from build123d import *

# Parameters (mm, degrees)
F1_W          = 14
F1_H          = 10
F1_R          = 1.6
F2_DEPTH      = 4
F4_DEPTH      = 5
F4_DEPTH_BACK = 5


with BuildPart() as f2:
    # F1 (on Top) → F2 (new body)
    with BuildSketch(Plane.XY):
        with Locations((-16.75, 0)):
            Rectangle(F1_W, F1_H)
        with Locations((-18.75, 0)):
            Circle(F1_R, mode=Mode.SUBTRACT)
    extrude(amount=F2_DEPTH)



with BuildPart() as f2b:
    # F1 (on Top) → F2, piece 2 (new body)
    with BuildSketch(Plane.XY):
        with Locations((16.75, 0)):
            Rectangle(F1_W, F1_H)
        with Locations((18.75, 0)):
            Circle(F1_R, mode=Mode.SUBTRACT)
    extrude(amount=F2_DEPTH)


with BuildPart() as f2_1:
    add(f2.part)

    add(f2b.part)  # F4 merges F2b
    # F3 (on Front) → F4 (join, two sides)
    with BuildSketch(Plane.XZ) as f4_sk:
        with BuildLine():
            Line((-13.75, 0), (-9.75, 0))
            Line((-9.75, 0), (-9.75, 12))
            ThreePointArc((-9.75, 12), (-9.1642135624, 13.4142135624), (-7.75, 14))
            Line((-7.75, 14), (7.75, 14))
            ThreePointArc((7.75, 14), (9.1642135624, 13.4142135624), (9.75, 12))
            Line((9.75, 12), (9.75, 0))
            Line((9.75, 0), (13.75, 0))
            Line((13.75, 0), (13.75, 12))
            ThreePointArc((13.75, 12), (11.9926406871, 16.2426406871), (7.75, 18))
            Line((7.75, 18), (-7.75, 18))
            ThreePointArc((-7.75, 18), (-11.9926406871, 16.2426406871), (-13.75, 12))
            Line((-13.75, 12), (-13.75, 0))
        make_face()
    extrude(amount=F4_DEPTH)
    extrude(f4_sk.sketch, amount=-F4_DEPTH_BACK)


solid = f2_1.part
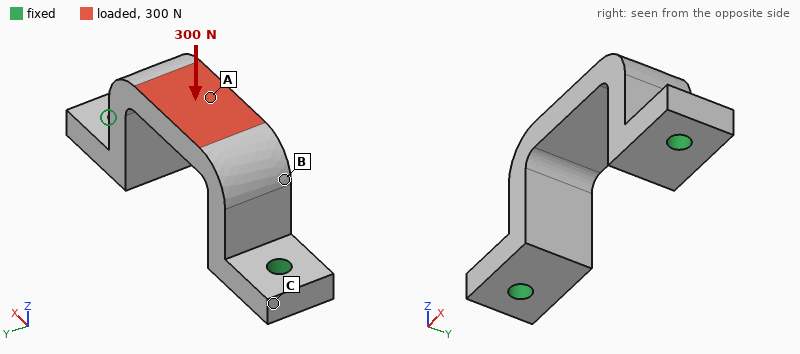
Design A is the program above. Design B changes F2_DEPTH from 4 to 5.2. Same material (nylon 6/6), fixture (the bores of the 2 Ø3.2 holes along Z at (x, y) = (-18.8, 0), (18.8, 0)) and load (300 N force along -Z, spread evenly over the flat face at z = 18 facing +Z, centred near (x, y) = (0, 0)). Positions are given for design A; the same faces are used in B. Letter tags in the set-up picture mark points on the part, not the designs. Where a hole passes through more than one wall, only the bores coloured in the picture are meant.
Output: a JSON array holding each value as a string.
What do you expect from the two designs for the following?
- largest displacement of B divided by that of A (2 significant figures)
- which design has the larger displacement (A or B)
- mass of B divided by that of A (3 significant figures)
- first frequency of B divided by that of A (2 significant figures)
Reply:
["0.90", "A", "1.08", "1.3"]
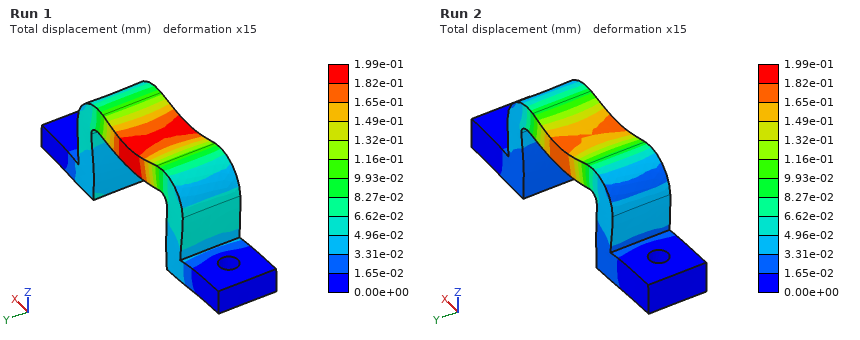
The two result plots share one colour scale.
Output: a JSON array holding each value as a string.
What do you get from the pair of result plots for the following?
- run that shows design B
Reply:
["Run 2"]
